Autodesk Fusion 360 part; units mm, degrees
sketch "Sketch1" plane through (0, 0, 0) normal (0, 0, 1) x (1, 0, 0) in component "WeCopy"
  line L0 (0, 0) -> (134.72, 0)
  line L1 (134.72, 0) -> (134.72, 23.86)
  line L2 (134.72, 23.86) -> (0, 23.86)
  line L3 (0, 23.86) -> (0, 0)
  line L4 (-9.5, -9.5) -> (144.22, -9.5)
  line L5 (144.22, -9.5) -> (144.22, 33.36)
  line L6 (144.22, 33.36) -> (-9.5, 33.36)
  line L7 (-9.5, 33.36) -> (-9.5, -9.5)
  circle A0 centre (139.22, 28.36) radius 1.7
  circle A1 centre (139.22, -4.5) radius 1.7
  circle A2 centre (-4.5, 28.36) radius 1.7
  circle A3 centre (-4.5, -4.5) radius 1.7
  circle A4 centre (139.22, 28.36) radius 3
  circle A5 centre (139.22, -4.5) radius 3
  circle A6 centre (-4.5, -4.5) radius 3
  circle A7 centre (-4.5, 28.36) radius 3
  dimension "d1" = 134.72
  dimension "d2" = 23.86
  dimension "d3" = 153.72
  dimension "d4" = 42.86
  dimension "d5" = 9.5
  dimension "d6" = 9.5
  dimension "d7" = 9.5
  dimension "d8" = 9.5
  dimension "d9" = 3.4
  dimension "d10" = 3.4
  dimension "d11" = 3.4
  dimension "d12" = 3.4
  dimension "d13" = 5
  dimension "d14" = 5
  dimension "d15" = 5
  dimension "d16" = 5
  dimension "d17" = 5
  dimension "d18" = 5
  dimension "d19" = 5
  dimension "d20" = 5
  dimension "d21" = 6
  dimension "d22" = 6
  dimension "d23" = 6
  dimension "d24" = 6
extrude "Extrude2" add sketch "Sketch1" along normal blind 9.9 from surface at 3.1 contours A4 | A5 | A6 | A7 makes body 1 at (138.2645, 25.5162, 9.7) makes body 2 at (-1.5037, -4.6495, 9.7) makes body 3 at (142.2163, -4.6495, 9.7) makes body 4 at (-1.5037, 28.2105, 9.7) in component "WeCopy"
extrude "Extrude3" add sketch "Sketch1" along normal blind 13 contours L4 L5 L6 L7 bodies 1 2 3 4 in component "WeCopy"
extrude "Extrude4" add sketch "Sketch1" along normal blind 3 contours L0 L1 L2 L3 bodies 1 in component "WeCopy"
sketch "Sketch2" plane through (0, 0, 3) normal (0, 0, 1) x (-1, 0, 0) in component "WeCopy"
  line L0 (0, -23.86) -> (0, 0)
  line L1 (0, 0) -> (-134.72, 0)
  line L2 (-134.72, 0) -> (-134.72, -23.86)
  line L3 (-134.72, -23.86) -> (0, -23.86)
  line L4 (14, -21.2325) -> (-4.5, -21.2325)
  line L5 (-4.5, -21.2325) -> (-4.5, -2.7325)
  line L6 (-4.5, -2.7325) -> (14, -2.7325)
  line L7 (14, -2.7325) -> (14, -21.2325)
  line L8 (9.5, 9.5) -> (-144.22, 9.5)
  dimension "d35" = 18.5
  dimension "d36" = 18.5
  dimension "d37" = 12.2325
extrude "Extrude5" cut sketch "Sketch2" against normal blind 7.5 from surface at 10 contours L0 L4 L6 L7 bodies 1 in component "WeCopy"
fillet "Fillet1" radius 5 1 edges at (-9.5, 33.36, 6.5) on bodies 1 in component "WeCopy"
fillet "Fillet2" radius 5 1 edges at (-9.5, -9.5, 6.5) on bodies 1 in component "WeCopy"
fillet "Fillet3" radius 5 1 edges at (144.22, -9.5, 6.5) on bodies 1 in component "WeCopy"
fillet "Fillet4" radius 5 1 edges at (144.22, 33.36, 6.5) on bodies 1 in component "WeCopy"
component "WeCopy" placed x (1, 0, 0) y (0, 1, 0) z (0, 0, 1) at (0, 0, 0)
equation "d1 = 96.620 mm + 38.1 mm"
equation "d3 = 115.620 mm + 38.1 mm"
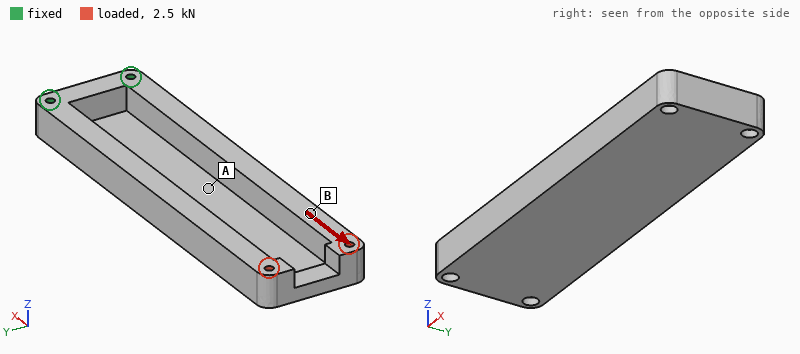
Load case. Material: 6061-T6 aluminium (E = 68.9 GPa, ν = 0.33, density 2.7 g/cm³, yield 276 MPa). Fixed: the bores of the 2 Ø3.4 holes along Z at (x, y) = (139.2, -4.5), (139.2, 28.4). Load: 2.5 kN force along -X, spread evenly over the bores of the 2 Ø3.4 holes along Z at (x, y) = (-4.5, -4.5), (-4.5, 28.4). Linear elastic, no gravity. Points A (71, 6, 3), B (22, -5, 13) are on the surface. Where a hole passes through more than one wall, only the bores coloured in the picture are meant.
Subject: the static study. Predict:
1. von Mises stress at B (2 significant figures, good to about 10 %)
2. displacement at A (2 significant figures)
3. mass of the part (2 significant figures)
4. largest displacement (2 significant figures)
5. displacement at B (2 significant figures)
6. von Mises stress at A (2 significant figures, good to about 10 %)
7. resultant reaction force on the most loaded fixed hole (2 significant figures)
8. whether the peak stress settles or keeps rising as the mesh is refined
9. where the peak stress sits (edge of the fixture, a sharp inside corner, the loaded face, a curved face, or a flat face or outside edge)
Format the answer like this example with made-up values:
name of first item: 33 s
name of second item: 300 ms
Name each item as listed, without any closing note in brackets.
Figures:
von Mises stress at B: 18 MPa
displacement at A: 0.040 mm
mass of the part: 140 g
largest displacement: 0.21 mm
displacement at B: 0.13 mm
von Mises stress at A: 4.6 MPa
resultant reaction force on the most loaded fixed hole: 1.3 kN
whether the peak stress settles or keeps rising as the mesh is refined: keeps rising
where the peak stress sits: edge of the fixture
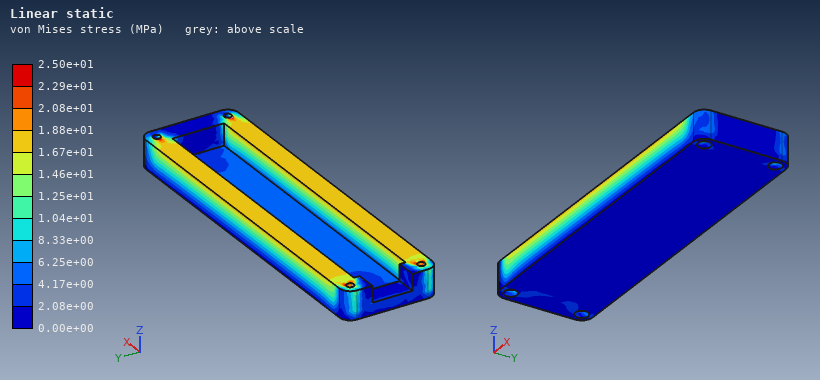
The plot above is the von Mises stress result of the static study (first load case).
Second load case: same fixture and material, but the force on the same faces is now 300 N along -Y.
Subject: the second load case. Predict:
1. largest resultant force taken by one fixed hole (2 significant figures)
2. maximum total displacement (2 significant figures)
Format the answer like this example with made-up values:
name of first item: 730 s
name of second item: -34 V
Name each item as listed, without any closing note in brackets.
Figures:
largest resultant force taken by one fixed hole: 1.2 kN
maximum total displacement: 0.14 mm
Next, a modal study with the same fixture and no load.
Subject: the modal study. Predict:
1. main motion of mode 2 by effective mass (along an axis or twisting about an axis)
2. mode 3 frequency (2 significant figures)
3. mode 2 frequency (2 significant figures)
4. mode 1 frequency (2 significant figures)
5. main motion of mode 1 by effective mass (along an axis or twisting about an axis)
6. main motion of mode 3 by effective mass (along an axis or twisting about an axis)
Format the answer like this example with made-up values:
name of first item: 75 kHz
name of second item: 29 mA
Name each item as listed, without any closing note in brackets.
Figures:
main motion of mode 2 by effective mass: along Y
mode 3 frequency: 2000 Hz
mode 2 frequency: 1200 Hz
mode 1 frequency: 450 Hz
main motion of mode 1 by effective mass: along Z
main motion of mode 3 by effective mass: along Y
